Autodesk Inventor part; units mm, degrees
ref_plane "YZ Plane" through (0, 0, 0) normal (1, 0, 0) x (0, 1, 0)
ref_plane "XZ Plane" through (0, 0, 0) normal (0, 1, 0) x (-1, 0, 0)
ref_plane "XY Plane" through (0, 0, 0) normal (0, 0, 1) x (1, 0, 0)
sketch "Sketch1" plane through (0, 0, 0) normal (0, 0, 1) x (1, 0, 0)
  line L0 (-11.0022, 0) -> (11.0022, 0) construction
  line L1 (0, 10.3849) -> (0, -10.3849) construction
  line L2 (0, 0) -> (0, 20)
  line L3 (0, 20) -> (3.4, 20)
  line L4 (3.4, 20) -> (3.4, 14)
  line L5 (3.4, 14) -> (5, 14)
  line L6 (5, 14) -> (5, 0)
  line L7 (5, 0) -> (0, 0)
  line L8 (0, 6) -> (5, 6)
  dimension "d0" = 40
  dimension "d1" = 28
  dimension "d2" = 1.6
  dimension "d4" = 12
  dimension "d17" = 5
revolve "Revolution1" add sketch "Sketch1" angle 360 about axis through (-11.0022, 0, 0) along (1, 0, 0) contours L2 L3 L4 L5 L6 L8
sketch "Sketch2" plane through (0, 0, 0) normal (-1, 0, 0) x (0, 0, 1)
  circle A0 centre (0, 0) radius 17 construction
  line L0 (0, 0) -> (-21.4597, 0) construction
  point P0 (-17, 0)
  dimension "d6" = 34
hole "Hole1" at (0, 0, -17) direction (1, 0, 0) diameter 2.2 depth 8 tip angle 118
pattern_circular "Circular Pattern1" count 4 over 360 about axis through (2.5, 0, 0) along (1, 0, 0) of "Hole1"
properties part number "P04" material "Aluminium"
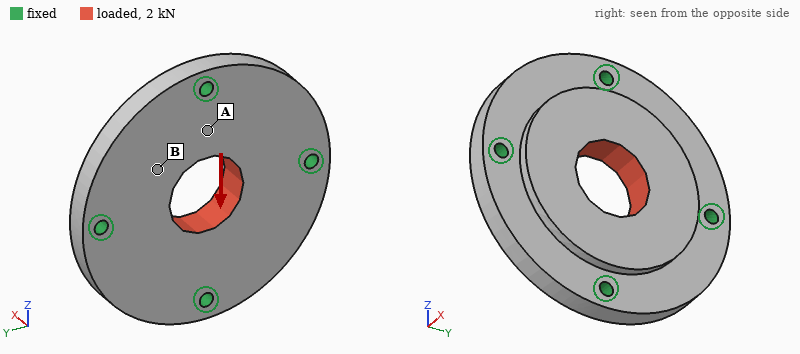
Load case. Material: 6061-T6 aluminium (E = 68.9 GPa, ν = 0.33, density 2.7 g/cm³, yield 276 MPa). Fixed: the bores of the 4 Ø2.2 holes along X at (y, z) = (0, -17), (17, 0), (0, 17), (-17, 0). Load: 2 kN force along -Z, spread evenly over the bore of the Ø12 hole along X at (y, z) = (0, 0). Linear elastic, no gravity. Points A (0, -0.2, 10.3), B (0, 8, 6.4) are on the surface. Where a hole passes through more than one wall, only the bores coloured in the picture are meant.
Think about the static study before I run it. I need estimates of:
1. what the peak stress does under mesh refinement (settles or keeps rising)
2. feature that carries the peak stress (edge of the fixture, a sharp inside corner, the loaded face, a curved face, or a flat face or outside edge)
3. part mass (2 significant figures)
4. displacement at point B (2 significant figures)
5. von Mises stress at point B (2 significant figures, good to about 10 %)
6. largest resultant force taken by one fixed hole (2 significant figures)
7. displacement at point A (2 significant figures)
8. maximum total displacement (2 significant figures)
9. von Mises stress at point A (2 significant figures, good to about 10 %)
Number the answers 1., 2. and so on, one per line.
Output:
1. keeps rising
2. edge of the fixture
3. 13 g
4. 2.5 µm
5. 8.3 MPa
6. 620 N
7. 1.9 µm
8. 3.6 µm
9. 18 MPa
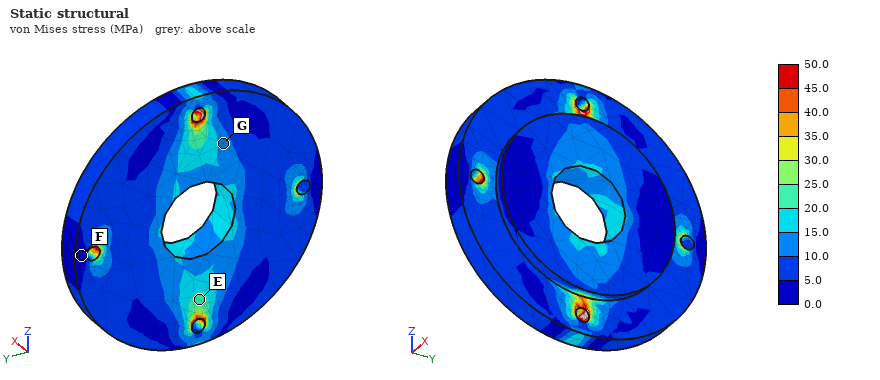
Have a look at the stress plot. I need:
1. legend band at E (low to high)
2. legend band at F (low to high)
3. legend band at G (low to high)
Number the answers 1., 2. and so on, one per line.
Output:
1. 20.0 to 25.0 MPa
2. 0.0 to 5.0 MPa
3. 10.0 to 15.0 MPa
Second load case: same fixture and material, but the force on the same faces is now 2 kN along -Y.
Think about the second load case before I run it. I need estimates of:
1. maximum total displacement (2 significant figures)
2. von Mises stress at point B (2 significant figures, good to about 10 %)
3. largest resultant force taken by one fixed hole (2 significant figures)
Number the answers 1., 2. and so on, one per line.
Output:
1. 3.6 µm
2. 10 MPa
3. 620 N
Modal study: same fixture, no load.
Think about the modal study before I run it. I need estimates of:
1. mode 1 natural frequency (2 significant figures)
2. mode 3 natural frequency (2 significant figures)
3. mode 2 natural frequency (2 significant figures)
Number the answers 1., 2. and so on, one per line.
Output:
1. 22 kHz
2. 25 kHz
3. 23 kHz
